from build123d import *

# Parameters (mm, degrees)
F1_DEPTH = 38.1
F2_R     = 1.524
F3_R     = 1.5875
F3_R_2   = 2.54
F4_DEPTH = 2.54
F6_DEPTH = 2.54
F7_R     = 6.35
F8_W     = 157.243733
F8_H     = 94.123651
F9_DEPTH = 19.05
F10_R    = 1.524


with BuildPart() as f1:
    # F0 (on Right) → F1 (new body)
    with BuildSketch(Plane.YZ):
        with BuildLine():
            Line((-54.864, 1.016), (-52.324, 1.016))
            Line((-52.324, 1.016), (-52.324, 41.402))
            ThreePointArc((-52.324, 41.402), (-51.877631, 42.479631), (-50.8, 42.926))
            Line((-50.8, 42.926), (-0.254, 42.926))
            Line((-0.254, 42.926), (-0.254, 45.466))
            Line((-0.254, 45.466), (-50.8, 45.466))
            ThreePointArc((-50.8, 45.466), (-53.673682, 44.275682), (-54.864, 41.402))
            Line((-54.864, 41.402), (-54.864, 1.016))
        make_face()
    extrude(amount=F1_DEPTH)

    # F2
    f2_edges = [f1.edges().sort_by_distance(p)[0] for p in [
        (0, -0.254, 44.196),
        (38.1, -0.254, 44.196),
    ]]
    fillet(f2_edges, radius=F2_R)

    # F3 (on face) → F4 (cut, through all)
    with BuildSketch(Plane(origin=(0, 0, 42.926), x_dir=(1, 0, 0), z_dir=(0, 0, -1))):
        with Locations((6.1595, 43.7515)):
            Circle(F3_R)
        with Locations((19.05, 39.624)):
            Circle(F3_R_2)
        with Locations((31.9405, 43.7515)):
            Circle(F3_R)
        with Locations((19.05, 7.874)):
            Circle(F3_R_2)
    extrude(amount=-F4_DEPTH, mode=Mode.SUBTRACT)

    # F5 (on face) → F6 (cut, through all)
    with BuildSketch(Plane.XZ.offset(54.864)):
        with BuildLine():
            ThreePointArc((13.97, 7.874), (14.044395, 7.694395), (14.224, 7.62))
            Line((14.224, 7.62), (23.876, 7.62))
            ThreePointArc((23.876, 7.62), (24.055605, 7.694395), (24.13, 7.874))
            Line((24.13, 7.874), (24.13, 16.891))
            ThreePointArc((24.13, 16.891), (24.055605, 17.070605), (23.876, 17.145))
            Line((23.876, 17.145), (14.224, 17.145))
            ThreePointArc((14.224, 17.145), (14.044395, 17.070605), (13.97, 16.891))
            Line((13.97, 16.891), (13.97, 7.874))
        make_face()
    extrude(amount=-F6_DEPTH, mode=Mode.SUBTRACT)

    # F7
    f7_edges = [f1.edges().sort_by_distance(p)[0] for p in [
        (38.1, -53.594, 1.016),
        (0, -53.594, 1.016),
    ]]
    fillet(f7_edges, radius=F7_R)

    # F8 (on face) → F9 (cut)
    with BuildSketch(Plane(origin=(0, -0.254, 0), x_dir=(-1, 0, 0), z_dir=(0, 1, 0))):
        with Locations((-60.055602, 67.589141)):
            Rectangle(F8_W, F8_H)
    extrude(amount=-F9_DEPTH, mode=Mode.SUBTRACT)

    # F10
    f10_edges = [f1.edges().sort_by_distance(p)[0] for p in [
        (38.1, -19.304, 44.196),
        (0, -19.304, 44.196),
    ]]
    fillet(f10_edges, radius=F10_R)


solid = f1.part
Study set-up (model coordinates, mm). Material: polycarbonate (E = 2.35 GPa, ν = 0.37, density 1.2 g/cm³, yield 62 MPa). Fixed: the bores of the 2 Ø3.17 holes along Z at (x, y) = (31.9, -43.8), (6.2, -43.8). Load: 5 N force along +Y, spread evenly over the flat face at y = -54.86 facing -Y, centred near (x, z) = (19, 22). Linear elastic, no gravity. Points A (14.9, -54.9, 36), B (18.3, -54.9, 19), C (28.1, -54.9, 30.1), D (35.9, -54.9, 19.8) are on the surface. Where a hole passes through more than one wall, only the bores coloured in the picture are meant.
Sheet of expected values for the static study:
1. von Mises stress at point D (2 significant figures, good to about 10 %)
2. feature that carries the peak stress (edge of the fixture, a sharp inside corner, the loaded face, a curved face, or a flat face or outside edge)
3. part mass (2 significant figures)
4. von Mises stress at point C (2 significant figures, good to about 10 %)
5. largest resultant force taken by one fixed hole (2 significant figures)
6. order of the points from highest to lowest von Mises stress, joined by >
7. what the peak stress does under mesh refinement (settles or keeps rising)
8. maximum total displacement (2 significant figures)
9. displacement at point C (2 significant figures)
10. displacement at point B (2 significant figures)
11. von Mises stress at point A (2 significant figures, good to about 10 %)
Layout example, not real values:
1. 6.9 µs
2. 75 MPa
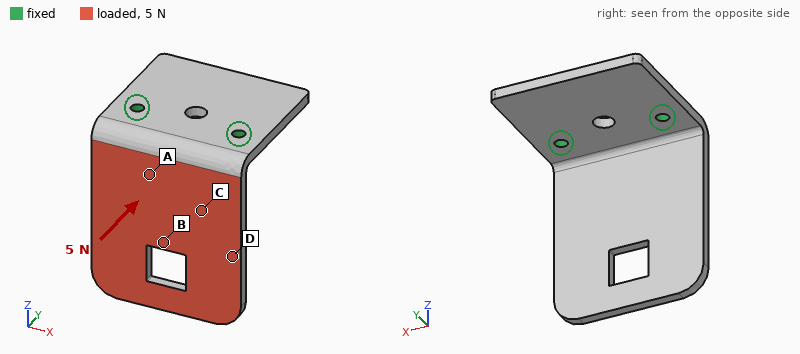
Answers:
1. 0.58 MPa
2. edge of the fixture
3. 8.4 g
4. 1.1 MPa
5. 2.6 N
6. A > C > D > B
7. keeps rising
8. 0.72 mm
9. 0.18 mm
10. 0.37 mm
11. 1.5 MPa
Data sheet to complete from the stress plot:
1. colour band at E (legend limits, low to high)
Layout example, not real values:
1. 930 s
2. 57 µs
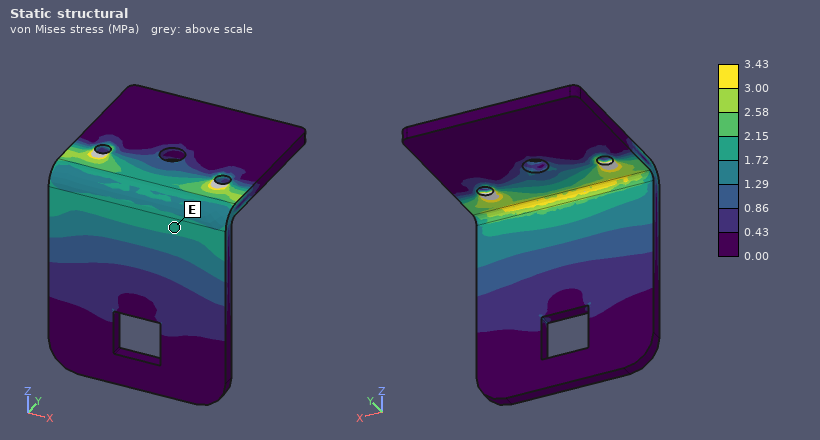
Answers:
1. 1.72 to 2.15 MPa
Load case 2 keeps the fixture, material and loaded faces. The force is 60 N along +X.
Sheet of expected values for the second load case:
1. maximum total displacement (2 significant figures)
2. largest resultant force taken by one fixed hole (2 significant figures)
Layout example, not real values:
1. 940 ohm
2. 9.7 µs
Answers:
1. 0.63 mm
2. 62 N
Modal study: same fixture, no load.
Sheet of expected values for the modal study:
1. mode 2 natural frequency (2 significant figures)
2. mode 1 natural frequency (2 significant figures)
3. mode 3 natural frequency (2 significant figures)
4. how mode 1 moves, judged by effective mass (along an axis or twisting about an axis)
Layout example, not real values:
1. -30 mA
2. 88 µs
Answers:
1. 680 Hz
2. 250 Hz
3. 920 Hz
4. along Y
